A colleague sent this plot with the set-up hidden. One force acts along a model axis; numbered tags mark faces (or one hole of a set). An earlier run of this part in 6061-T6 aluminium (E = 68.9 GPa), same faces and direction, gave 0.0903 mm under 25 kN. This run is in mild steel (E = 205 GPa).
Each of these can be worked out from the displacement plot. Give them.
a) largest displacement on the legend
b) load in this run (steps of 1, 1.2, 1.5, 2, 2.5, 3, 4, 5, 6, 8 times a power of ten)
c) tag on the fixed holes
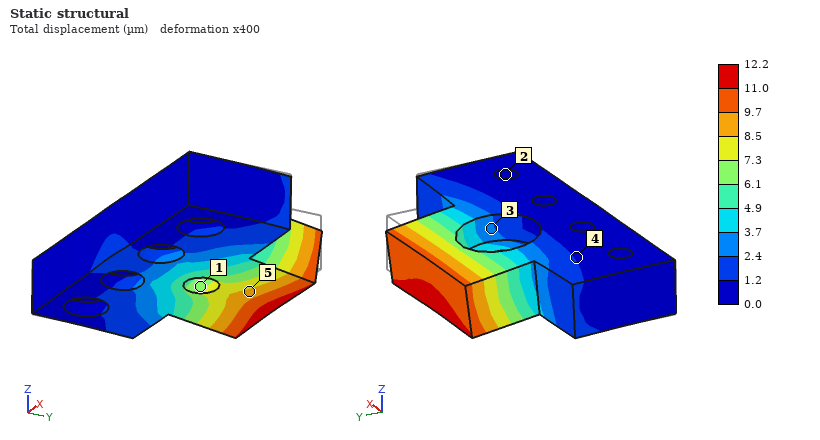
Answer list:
12.2 µm
10 kN
2
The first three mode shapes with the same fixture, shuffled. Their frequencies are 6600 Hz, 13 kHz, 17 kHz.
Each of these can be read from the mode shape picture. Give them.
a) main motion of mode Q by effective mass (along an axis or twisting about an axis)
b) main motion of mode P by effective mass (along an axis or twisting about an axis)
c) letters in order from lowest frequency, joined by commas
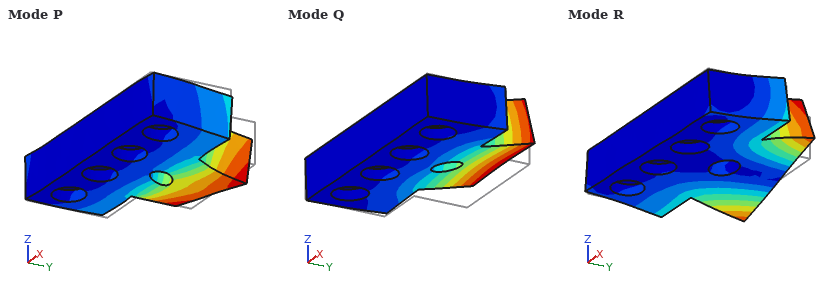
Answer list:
along Z
along X
Q, R, P
